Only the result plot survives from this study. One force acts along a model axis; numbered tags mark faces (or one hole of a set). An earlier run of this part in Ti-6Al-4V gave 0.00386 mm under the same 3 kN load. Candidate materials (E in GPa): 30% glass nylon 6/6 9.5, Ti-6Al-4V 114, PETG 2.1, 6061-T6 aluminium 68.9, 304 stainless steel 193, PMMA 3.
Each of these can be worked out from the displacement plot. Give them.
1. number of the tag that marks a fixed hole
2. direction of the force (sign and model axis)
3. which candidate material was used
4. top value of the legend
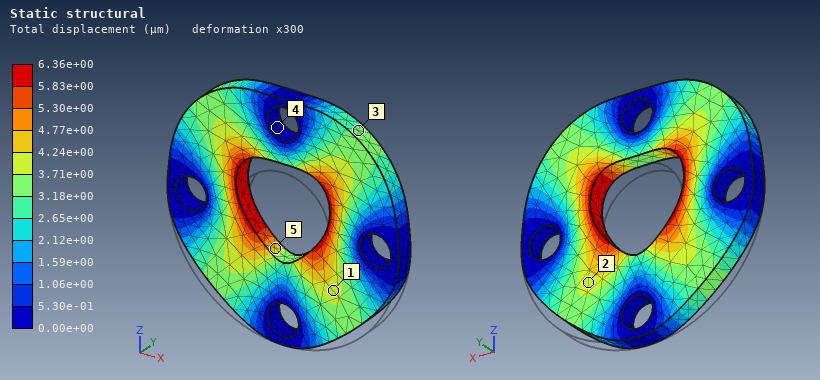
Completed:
4
+Z
6061-T6 aluminium
6.36e+00 µm
